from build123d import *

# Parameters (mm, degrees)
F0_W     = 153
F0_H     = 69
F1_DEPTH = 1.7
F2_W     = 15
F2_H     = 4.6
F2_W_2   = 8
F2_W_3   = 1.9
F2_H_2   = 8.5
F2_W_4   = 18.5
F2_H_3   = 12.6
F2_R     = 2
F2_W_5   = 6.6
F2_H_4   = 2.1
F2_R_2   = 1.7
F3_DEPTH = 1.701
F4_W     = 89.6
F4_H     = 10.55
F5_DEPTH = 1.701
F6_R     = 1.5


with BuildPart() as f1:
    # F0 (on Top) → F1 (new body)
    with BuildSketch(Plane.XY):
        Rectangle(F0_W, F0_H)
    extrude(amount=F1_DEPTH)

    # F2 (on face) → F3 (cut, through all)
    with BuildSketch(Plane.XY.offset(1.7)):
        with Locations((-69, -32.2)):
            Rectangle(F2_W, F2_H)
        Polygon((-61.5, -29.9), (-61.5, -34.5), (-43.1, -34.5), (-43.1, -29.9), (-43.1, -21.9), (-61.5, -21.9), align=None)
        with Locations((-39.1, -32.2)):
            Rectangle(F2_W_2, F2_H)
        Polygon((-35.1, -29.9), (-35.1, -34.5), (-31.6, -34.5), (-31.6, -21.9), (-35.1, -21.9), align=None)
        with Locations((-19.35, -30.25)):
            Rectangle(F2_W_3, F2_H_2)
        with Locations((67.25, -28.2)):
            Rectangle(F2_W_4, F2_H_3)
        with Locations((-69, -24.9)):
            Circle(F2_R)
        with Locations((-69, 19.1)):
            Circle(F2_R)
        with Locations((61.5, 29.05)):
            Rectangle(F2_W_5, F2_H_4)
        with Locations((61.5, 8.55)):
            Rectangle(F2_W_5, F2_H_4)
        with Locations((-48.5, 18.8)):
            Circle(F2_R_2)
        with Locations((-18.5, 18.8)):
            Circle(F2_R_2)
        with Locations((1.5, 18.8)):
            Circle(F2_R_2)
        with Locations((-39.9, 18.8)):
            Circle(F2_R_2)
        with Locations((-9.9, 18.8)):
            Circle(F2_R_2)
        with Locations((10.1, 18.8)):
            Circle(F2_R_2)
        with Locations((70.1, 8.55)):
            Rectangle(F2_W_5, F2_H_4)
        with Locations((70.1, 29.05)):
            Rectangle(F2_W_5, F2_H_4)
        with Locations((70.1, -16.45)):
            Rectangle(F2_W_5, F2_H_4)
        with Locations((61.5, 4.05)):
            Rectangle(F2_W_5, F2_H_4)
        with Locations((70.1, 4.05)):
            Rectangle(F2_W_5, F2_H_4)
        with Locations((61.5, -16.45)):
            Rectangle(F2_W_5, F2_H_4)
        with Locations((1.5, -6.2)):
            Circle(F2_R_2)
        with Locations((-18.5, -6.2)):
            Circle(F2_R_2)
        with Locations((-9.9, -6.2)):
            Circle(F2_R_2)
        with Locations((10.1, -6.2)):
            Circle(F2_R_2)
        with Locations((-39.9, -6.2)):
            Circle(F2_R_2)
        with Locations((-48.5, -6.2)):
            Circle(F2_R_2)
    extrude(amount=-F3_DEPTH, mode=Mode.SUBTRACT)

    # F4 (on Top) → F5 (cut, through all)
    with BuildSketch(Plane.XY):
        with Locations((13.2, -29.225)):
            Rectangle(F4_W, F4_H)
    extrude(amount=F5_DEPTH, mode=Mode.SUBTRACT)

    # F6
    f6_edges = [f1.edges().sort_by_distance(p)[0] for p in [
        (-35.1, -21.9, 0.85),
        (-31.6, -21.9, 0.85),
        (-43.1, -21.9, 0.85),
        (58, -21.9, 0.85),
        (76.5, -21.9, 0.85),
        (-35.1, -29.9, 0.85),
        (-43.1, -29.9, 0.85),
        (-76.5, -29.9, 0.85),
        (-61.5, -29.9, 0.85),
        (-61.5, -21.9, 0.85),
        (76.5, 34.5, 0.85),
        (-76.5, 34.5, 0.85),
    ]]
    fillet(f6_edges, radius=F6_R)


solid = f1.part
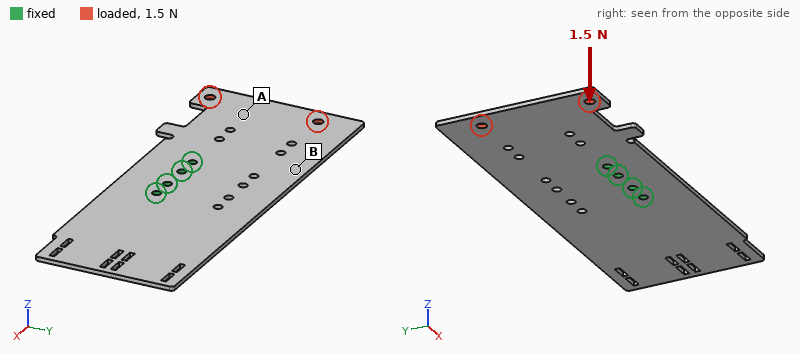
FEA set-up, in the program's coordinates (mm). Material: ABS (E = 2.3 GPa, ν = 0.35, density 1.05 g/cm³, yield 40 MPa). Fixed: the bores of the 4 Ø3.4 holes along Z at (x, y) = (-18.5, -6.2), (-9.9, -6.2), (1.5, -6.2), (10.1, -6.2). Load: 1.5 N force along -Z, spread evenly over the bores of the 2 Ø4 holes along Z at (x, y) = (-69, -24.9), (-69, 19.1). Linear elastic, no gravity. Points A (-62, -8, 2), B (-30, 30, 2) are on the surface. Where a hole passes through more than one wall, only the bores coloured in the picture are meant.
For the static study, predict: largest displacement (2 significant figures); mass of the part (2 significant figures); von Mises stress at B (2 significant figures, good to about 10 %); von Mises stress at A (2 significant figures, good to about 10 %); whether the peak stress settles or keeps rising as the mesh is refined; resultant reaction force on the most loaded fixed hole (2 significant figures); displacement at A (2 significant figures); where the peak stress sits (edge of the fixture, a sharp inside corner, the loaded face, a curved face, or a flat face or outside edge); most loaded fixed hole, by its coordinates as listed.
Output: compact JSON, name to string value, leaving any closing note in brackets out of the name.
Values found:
{"largest displacement": "1.8 mm", "mass of the part": "16 g", "von Mises stress at B": "1.4 MPa", "von Mises stress at A": "0.59 MPa", "whether the peak stress settles or keeps rising as the mesh is refined": "keeps rising", "resultant reaction force on the most loaded fixed hole": "4.7 N", "displacement at A": "1.1 mm", "where the peak stress sits": "edge of the fixture", "most loaded fixed hole, by its coordinates as listed": "(-18.5, -6.2)"}
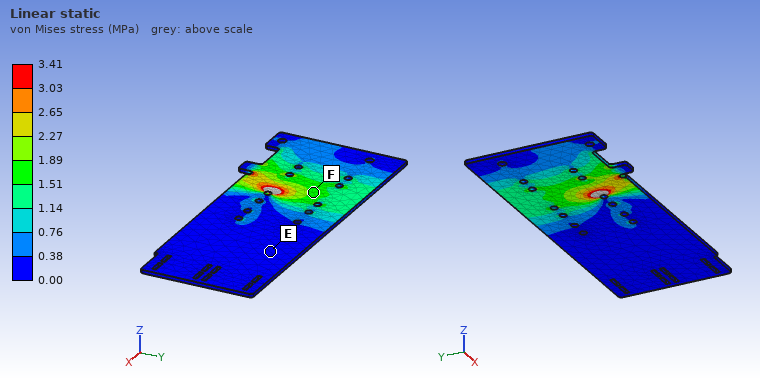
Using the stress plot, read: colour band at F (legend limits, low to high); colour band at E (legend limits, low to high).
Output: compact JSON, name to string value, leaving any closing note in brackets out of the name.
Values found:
{"colour band at F": "1.51 to 1.89 MPa", "colour band at E": "0.00 to 0.38 MPa"}
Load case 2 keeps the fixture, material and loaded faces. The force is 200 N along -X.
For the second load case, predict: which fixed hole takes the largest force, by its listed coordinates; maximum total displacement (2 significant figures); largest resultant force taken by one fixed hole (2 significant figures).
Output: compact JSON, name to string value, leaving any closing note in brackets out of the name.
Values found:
{"which fixed hole takes the largest force, by its listed coordinates": "(-18.5, -6.2)", "maximum total displacement": "0.22 mm", "largest resultant force taken by one fixed hole": "110 N"}
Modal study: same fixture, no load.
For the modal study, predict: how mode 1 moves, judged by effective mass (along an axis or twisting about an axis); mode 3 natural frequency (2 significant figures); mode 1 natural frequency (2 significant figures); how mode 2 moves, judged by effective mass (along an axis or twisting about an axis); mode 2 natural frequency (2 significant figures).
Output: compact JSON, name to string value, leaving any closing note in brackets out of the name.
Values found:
{"how mode 1 moves, judged by effective mass": "along Z", "mode 3 natural frequency": "170 Hz", "mode 1 natural frequency": "86 Hz", "how mode 2 moves, judged by effective mass": "along Z", "mode 2 natural frequency": "100 Hz"}
